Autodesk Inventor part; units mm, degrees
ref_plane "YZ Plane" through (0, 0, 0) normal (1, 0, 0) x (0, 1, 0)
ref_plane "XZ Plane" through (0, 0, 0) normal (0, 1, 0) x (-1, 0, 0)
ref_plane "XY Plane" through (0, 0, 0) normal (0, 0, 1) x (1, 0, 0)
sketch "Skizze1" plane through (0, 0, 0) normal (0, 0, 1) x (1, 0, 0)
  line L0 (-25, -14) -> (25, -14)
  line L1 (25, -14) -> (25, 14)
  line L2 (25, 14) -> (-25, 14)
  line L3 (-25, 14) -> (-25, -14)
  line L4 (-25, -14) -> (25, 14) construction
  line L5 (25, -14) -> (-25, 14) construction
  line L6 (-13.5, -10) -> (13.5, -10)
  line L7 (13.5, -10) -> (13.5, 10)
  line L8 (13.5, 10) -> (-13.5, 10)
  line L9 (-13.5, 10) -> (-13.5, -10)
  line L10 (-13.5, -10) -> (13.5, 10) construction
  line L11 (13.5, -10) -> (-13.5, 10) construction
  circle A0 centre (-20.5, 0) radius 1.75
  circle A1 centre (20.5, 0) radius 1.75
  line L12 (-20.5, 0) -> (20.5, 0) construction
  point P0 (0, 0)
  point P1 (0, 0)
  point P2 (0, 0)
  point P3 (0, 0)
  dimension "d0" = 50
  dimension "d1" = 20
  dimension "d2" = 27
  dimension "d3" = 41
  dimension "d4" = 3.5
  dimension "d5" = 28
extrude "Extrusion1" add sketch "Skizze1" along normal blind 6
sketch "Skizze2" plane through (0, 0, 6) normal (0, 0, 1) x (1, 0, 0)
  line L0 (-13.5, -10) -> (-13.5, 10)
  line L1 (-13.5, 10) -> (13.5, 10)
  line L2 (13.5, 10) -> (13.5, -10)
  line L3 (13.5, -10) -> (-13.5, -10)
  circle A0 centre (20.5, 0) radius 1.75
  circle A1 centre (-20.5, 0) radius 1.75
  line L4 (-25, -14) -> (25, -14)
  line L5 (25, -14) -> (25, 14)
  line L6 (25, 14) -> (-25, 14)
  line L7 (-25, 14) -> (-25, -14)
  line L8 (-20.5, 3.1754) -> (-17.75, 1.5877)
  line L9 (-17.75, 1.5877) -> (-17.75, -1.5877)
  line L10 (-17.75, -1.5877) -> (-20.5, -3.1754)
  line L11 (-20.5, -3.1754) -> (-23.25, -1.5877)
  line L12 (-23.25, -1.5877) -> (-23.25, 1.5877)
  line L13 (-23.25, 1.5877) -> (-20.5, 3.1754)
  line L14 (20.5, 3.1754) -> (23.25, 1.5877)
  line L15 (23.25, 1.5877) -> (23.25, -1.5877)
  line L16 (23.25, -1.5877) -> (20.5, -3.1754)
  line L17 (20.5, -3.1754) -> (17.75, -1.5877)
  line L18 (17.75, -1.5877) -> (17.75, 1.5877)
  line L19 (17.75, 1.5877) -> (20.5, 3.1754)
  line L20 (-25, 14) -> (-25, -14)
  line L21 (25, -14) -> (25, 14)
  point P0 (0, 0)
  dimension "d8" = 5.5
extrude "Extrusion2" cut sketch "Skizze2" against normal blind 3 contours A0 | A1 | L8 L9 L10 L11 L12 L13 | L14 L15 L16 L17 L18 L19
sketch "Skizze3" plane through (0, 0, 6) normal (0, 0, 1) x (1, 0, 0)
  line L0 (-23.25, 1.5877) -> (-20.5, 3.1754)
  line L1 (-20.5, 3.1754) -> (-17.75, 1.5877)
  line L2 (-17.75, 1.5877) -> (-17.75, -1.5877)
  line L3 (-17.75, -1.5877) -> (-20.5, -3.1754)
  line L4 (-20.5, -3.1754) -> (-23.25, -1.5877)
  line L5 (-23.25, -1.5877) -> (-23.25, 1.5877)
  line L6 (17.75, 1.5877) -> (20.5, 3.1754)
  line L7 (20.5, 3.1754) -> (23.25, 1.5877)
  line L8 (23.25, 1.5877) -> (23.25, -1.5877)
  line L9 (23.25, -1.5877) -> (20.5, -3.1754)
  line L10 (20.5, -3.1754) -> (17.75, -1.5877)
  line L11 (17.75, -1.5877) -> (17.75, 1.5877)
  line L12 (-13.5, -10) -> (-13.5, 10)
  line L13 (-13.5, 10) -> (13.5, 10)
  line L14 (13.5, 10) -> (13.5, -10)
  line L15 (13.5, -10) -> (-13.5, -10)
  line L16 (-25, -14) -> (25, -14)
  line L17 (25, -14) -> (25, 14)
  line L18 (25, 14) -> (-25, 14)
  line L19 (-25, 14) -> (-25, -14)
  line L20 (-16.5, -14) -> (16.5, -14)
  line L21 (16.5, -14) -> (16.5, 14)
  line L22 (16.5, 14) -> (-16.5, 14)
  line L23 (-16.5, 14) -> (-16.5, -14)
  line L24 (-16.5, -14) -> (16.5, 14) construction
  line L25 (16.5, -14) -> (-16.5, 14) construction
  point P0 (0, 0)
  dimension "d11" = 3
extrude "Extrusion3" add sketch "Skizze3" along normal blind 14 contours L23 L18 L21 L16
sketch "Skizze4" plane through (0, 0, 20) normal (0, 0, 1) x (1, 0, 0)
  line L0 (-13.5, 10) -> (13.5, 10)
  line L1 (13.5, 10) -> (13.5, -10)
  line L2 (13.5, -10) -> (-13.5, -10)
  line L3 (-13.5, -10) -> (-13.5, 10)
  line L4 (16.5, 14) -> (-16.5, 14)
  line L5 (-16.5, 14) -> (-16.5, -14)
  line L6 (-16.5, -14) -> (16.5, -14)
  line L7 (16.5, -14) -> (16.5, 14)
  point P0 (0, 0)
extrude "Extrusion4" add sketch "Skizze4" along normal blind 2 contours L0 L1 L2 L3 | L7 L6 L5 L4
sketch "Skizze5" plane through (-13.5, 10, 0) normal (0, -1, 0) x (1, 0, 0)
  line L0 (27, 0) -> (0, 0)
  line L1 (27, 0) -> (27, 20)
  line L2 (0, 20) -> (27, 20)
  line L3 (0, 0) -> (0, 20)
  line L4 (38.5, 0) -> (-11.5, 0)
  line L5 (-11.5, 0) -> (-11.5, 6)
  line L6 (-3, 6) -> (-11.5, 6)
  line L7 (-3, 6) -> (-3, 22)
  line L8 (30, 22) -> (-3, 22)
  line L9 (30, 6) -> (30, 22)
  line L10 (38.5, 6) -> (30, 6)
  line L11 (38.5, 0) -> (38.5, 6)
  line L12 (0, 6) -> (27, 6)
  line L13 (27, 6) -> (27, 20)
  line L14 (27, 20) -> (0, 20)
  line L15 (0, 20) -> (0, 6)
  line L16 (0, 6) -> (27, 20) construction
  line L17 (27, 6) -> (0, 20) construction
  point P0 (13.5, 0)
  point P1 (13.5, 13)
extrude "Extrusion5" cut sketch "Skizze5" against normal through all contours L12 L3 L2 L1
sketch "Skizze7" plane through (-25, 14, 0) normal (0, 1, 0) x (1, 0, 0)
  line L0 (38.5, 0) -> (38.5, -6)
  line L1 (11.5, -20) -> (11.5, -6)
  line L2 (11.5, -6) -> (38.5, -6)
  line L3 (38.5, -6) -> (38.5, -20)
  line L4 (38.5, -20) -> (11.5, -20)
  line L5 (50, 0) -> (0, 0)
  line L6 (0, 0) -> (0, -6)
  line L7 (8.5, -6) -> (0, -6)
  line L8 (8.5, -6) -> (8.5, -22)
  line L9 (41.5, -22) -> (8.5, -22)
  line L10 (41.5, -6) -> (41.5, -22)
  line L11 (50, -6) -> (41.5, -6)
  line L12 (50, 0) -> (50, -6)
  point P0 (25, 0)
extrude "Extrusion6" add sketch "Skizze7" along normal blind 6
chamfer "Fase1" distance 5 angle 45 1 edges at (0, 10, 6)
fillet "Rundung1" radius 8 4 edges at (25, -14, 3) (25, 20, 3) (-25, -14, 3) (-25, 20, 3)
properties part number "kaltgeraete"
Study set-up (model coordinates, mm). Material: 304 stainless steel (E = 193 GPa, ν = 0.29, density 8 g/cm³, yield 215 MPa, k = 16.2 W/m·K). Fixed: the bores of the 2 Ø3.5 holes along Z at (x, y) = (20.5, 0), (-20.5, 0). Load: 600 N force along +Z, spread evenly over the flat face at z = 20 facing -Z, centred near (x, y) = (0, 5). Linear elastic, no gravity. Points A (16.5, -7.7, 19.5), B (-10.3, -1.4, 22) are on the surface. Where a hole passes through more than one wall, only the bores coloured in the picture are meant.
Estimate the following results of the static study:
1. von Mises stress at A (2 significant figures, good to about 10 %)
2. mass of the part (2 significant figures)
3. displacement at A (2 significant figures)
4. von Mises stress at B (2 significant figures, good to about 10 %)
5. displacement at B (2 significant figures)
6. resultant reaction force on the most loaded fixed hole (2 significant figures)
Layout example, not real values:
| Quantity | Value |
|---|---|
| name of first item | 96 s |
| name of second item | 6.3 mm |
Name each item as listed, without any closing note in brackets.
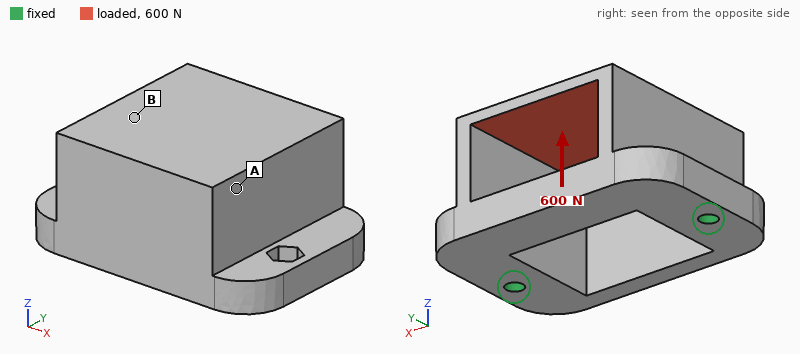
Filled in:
| Quantity | Value |
|---|---|
| von Mises stress at A | 6.6 MPa |
| mass of the part | 100 g |
| displacement at A | 5.6 µm |
| von Mises stress at B | 18 MPa |
| displacement at B | 7.0 µm |
| resultant reaction force on the most loaded fixed hole | 320 N |
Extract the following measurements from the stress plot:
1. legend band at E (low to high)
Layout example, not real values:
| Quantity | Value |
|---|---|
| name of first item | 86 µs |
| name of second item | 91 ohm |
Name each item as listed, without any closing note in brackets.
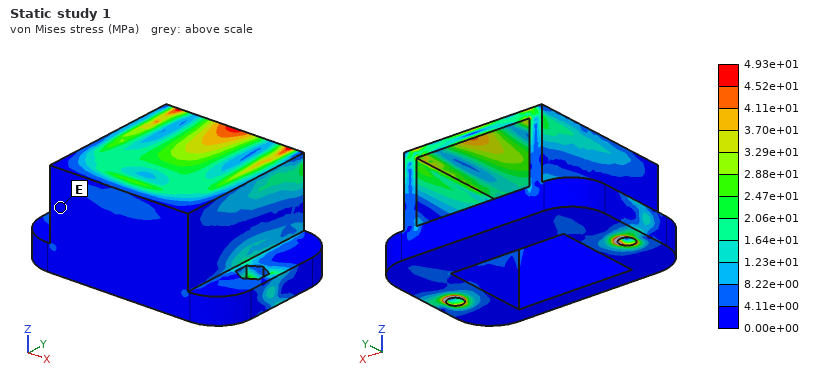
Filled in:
| Quantity | Value |
|---|---|
| legend band at E | 0.00e+00 to 4.11e+00 MPa |
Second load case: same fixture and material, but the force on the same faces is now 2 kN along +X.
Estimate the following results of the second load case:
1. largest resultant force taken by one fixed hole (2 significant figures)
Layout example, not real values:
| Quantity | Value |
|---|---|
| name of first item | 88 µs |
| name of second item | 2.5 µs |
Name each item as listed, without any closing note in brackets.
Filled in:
| Quantity | Value |
|---|---|
| largest resultant force taken by one fixed hole | 1.3 kN |
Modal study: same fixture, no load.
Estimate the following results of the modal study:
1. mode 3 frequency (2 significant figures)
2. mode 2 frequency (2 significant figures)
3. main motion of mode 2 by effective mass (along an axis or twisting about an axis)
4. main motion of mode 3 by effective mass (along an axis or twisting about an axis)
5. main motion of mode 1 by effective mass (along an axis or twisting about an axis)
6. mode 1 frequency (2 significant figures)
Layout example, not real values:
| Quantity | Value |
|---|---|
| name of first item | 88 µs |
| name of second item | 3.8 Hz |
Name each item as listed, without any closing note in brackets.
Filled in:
| Quantity | Value |
|---|---|
| mode 3 frequency | 11 kHz |
| mode 2 frequency | 6600 Hz |
| main motion of mode 2 by effective mass | along X |
| main motion of mode 3 by effective mass | along Z |
| main motion of mode 1 by effective mass | along Y |
| mode 1 frequency | 3100 Hz |
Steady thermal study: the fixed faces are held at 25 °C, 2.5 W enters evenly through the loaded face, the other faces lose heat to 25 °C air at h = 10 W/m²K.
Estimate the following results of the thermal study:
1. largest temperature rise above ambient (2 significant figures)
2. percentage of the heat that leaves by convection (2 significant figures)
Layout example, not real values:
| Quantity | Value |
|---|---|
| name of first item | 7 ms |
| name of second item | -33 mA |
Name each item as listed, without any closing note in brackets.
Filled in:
| Quantity | Value |
|---|---|
| largest temperature rise above ambient | 23 K |
| percentage of the heat that leaves by convection | 26 % |
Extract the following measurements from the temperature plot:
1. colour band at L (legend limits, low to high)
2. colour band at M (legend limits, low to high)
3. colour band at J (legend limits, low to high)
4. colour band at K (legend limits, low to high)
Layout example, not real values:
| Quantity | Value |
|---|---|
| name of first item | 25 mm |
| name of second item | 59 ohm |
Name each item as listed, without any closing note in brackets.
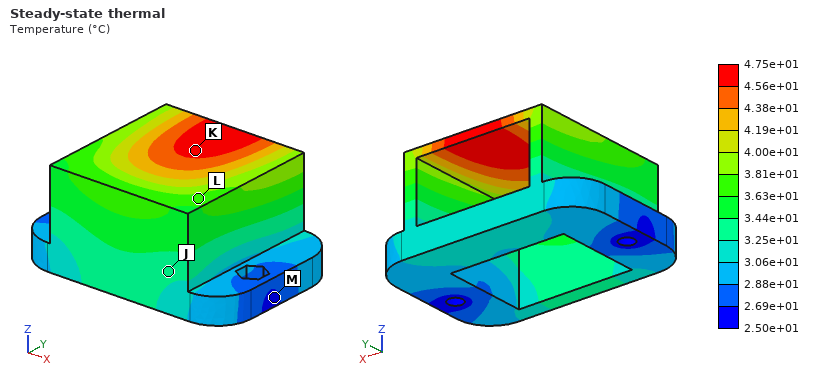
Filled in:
| Quantity | Value |
|---|---|
| colour band at L | 3.63e+01 to 3.81e+01 °C |
| colour band at M | 2.50e+01 to 2.69e+01 °C |
| colour band at J | 3.25e+01 to 3.44e+01 °C |
| colour band at K | 4.56e+01 to 4.75e+01 °C |
